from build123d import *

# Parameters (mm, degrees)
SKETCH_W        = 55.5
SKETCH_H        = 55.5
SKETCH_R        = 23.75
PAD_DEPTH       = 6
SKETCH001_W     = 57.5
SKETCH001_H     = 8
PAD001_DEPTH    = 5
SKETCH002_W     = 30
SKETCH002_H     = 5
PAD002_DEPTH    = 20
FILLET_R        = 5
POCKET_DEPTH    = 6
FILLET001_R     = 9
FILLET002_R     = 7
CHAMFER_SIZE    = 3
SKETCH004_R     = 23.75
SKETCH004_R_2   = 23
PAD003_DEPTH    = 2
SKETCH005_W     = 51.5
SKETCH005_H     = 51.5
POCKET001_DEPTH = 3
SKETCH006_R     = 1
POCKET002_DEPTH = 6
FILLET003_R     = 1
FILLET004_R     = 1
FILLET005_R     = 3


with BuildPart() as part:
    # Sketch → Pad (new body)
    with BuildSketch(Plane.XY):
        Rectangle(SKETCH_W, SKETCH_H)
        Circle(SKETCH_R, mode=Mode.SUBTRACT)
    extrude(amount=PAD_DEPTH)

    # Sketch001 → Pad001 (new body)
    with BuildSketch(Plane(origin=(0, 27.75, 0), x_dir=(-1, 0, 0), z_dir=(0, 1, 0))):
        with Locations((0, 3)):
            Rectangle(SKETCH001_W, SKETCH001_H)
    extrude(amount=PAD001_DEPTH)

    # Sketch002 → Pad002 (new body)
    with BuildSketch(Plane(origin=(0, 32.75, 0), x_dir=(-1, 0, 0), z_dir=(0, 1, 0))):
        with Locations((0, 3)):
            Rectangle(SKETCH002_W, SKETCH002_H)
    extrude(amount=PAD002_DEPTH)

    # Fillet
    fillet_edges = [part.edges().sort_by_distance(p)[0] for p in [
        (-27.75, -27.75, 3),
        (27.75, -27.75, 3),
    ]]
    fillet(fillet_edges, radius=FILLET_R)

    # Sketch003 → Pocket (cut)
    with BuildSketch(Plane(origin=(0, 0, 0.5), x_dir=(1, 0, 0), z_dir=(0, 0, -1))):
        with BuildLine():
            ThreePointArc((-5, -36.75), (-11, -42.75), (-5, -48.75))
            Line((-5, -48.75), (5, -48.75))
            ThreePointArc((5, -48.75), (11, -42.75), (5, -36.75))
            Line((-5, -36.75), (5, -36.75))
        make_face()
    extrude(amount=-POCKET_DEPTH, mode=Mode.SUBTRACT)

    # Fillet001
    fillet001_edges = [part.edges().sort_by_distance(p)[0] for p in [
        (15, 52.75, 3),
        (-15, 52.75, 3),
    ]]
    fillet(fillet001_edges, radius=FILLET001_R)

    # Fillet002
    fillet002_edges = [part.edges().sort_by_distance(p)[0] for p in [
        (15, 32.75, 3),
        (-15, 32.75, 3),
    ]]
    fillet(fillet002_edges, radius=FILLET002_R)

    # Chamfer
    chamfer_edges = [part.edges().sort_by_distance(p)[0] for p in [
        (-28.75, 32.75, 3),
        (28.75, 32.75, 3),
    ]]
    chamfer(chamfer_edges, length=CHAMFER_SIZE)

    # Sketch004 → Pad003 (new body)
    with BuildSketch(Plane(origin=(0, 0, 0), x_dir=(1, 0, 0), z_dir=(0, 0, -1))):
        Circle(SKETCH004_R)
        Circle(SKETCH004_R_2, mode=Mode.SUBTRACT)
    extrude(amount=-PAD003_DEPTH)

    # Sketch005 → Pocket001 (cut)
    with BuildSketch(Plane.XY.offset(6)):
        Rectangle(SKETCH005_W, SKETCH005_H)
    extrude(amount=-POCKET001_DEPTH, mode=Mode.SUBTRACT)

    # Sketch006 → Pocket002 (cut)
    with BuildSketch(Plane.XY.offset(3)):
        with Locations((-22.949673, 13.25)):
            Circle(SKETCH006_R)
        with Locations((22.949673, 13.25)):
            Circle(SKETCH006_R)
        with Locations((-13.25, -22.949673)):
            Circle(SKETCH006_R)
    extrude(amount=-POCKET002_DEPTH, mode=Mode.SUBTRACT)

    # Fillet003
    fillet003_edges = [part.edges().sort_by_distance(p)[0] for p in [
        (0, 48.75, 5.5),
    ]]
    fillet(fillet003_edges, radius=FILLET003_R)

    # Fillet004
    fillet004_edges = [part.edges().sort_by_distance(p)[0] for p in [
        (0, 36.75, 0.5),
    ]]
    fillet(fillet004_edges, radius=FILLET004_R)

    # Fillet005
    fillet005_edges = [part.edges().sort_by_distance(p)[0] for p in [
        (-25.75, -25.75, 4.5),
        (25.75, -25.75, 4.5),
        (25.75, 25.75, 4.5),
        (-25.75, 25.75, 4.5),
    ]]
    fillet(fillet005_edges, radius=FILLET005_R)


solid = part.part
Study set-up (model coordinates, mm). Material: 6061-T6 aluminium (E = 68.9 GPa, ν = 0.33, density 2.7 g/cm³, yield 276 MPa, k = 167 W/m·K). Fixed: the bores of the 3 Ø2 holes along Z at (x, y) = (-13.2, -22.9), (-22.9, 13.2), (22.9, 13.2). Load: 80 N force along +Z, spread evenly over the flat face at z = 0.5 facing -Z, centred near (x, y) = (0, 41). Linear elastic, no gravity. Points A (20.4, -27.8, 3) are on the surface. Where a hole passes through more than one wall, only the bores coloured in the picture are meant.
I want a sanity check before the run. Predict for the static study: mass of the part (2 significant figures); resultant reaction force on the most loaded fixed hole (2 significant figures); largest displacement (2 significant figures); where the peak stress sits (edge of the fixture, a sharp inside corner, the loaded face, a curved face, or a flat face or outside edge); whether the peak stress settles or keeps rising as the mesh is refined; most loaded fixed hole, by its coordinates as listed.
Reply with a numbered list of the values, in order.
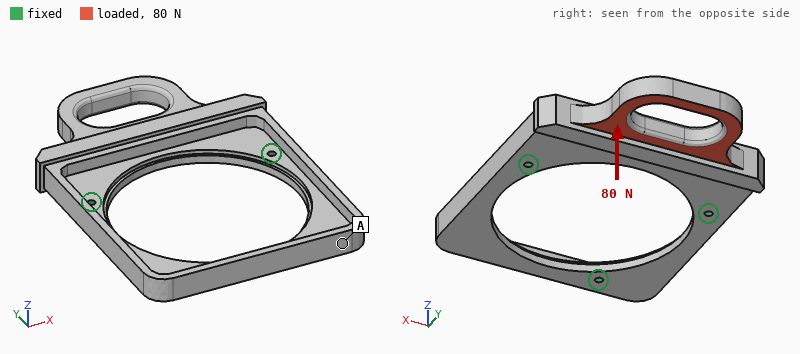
1. 25 g
2. 56 N
3. 0.14 mm
4. edge of the fixture
5. keeps rising
6. (-22.9, 13.2)
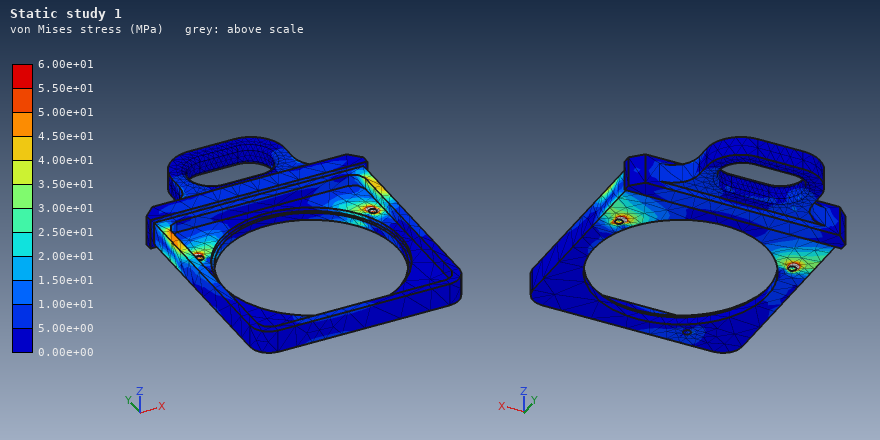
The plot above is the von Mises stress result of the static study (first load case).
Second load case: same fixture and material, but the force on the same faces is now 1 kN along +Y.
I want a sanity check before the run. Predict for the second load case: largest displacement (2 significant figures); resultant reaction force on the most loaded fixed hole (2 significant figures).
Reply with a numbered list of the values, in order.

1. 0.11 mm
2. 560 N
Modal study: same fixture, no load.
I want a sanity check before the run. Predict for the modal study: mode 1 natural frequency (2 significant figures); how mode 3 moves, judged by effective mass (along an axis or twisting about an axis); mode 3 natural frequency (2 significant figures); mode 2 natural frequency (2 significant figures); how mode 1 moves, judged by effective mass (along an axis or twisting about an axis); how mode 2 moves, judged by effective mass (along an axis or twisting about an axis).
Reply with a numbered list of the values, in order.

1. 1800 Hz
2. twisting about Y
3. 6400 Hz
4. 2600 Hz
5. along Z
6. along Z
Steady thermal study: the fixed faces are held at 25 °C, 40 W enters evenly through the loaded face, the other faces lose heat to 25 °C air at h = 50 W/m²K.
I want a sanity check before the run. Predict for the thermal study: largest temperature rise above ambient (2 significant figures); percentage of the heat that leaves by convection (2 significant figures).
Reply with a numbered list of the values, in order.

1. 82 K
2. 19 %
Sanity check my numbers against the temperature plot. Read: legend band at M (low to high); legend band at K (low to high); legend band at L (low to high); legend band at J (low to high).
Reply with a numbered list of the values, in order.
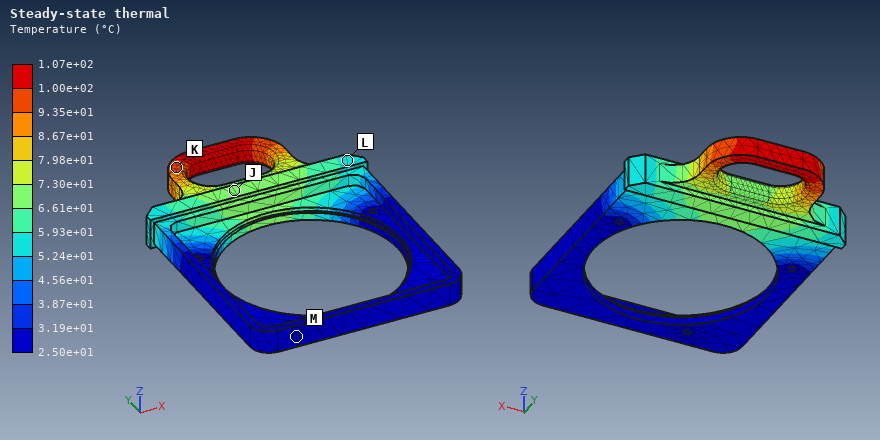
1. 2.50e+01 to 3.19e+01 °C
2. 9.35e+01 to 1.00e+02 °C
3. 5.24e+01 to 5.93e+01 °C
4. 6.61e+01 to 7.30e+01 °C
